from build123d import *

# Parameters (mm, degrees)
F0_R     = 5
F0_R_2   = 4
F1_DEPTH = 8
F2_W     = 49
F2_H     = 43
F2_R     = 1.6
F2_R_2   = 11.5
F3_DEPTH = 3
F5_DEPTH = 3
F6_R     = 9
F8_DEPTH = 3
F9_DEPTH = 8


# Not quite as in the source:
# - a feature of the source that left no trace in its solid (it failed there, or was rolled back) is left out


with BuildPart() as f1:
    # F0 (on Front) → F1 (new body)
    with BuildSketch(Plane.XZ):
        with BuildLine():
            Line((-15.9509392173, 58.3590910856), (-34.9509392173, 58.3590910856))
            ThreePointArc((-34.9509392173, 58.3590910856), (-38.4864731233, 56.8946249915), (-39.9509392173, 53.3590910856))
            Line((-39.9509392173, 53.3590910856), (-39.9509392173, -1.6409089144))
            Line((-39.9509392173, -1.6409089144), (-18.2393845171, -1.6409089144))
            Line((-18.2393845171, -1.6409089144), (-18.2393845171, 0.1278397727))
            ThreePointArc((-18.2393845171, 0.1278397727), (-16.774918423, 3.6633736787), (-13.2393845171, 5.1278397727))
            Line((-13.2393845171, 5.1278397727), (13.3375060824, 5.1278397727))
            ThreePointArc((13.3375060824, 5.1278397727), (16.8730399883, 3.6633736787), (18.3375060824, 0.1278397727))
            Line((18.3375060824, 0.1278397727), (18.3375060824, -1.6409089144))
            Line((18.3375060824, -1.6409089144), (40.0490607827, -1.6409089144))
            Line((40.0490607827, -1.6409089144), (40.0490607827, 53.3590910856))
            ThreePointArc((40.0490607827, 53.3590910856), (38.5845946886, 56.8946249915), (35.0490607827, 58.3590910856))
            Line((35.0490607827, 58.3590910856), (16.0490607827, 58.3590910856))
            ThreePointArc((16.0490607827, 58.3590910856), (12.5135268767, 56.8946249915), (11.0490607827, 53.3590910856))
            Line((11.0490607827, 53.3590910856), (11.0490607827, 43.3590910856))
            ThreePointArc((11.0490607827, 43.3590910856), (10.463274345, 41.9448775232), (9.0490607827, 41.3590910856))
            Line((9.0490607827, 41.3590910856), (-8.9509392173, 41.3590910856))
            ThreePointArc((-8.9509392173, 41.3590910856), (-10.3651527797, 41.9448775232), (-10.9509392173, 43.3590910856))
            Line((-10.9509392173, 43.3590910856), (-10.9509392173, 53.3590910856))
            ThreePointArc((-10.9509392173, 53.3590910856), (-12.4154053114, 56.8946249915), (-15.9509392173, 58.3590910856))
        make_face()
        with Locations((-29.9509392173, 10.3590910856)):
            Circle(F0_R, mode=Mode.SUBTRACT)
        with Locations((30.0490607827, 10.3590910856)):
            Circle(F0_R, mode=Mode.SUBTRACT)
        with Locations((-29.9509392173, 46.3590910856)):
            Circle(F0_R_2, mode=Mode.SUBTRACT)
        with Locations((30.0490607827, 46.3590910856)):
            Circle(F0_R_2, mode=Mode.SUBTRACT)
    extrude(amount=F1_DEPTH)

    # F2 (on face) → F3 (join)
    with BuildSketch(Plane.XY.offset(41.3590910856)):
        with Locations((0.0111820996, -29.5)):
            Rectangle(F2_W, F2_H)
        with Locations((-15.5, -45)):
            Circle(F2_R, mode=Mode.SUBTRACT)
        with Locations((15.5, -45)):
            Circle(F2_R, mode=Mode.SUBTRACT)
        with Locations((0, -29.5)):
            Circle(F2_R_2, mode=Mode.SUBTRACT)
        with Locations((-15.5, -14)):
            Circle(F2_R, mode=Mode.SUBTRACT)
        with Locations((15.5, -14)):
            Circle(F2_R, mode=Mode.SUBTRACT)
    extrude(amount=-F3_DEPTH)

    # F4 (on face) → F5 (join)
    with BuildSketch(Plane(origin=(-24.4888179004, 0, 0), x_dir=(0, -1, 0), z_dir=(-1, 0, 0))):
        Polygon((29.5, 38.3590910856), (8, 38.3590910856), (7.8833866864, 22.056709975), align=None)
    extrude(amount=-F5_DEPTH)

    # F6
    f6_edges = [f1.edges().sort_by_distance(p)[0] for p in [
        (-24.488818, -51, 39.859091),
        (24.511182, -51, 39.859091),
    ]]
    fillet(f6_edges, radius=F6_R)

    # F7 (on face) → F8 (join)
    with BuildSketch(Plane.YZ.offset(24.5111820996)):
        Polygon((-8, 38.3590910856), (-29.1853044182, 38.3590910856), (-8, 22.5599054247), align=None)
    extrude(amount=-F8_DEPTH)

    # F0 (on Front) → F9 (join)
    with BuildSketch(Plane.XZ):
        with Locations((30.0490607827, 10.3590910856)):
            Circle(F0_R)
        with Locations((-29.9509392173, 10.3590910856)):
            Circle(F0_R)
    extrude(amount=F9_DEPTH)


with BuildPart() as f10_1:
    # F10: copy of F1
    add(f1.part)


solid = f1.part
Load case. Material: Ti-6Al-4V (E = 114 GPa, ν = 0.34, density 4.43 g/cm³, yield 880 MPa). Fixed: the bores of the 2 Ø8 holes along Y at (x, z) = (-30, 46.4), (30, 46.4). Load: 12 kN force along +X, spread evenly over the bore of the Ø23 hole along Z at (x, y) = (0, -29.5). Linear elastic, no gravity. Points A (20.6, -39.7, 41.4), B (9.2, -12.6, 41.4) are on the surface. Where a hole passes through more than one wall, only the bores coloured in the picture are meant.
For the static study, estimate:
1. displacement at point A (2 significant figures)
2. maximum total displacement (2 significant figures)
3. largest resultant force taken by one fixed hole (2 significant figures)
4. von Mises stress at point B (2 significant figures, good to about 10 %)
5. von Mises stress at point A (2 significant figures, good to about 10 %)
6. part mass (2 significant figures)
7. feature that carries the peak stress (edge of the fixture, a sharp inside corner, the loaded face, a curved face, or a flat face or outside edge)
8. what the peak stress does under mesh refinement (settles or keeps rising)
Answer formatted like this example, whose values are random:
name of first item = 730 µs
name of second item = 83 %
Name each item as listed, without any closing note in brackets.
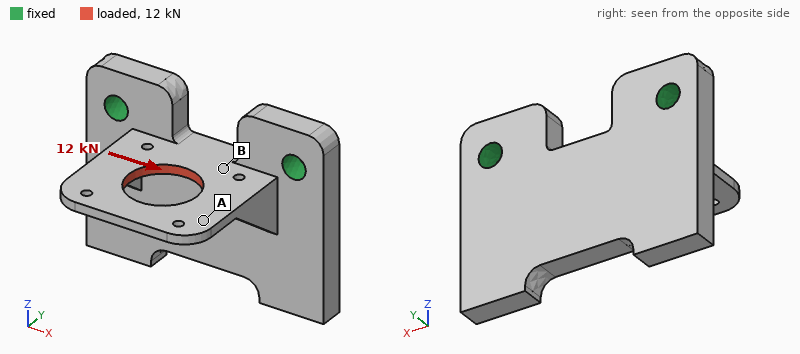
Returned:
displacement at point A = 0.18 mm
maximum total displacement = 0.22 mm
largest resultant force taken by one fixed hole = 8.4 kN
von Mises stress at point B = 160 MPa
von Mises stress at point A = 66 MPa
part mass = 170 g
feature that carries the peak stress = a sharp inside corner
what the peak stress does under mesh refinement = keeps rising
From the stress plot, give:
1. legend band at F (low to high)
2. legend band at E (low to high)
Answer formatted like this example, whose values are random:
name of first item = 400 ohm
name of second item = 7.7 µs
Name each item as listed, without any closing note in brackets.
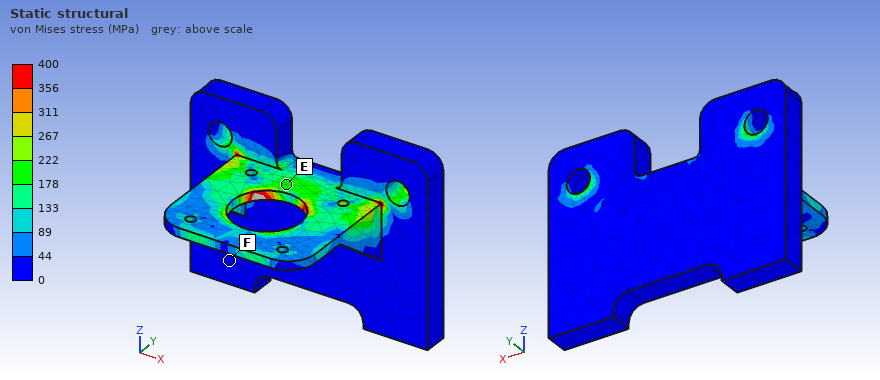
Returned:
legend band at F = 0 to 44 MPa
legend band at E = 178 to 222 MPa
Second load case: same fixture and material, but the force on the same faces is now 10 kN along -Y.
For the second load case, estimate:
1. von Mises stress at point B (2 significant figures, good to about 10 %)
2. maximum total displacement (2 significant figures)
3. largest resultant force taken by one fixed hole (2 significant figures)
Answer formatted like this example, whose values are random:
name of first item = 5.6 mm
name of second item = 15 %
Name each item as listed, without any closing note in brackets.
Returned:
von Mises stress at point B = 69 MPa
maximum total displacement = 76 µm
largest resultant force taken by one fixed hole = 5.2 kN
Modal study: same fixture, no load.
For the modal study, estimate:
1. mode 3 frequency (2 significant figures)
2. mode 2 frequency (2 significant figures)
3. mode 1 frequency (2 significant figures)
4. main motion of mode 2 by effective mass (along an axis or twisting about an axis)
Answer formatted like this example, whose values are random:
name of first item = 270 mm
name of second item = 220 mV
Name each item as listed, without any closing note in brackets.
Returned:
mode 3 frequency = 4400 Hz
mode 2 frequency = 3100 Hz
mode 1 frequency = 2100 Hz
main motion of mode 2 by effective mass = along Y
